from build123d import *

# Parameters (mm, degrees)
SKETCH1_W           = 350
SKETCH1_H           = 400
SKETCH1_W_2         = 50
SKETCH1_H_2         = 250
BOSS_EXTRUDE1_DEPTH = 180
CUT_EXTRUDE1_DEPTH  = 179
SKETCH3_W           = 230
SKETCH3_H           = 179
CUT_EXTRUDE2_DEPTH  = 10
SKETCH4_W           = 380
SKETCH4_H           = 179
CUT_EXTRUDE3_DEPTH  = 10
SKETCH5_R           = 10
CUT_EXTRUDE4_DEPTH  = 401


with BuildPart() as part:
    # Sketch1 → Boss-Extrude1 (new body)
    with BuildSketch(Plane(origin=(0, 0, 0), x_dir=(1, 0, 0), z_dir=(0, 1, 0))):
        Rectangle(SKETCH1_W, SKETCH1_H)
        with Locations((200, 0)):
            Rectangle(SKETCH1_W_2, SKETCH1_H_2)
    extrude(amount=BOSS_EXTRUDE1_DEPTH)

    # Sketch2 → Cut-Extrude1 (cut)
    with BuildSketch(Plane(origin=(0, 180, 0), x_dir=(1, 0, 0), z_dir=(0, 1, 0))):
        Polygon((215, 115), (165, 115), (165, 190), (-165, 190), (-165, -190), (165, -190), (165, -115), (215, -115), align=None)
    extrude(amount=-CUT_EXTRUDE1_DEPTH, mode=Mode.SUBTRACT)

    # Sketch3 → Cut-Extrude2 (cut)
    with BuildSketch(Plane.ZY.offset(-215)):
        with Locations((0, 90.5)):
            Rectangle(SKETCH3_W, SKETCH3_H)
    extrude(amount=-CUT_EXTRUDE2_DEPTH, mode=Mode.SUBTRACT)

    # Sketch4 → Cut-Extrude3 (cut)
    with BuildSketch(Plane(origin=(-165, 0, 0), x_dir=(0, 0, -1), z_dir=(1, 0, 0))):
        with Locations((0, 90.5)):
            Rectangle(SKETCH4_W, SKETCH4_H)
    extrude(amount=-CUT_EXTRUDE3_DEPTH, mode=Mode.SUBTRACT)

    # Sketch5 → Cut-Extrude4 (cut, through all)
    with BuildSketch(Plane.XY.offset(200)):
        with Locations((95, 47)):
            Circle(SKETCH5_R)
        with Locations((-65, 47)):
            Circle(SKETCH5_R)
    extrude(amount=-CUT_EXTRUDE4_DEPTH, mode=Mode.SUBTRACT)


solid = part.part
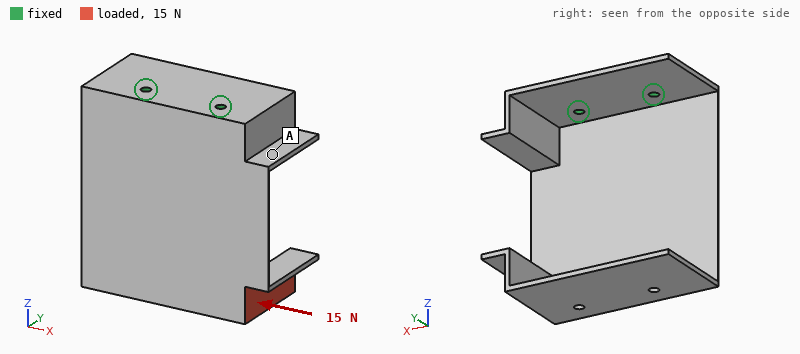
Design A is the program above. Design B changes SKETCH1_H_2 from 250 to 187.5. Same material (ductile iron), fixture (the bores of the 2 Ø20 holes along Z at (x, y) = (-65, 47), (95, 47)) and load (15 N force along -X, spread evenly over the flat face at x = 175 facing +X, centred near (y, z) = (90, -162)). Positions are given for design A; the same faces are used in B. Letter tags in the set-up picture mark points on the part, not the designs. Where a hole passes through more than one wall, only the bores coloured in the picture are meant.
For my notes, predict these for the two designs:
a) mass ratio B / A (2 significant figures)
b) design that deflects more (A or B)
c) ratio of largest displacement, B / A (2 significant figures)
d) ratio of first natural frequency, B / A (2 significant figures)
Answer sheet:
0.90
B
1.2
0.95
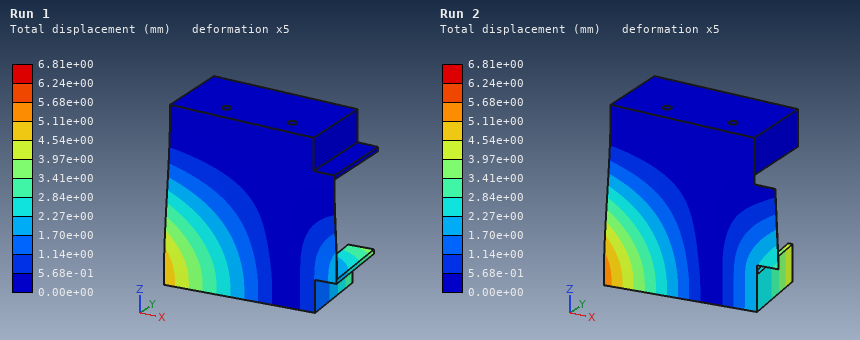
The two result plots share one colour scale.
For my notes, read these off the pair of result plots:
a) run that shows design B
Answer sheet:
Run 2
